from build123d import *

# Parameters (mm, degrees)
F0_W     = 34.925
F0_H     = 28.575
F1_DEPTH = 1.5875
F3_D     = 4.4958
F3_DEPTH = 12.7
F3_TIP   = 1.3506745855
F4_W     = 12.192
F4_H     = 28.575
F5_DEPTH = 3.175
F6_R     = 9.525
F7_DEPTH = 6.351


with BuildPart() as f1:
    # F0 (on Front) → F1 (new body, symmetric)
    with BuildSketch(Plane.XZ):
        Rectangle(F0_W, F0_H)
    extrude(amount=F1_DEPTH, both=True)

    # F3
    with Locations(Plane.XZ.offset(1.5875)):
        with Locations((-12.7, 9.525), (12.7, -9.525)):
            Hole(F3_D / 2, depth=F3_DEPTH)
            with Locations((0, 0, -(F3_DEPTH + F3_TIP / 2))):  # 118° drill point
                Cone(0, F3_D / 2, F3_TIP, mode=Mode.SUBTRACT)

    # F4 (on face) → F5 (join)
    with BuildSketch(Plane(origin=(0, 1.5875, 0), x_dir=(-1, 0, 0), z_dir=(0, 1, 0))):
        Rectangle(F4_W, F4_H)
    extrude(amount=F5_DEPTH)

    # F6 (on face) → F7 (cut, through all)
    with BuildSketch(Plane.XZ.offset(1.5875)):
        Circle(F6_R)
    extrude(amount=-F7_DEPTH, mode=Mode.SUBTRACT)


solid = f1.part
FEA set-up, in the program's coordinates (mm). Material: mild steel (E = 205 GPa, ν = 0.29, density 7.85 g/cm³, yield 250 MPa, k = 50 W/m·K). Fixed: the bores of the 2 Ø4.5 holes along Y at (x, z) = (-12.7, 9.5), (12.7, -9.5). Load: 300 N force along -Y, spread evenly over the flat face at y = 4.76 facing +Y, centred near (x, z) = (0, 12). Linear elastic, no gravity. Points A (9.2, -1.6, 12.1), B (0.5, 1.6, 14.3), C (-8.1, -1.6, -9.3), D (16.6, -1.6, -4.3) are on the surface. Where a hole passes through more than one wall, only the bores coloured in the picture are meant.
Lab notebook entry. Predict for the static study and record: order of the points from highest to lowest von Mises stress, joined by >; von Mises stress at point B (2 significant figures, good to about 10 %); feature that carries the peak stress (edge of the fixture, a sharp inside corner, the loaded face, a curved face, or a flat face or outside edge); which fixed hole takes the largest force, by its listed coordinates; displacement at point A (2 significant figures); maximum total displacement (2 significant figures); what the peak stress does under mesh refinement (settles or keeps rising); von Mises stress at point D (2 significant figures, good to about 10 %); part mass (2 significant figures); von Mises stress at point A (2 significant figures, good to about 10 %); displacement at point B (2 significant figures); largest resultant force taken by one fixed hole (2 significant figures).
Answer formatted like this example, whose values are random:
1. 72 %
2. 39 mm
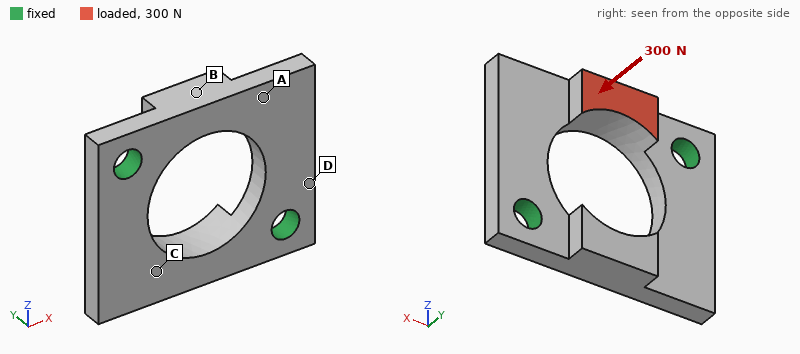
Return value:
1. D > A > B > C
2. 22 MPa
3. edge of the fixture
4. (-12.7, 9.5)
5. 21 µm
6. 27 µm
7. keeps rising
8. 48 MPa
9. 20 g
10. 31 MPa
11. 15 µm
12. 230 N
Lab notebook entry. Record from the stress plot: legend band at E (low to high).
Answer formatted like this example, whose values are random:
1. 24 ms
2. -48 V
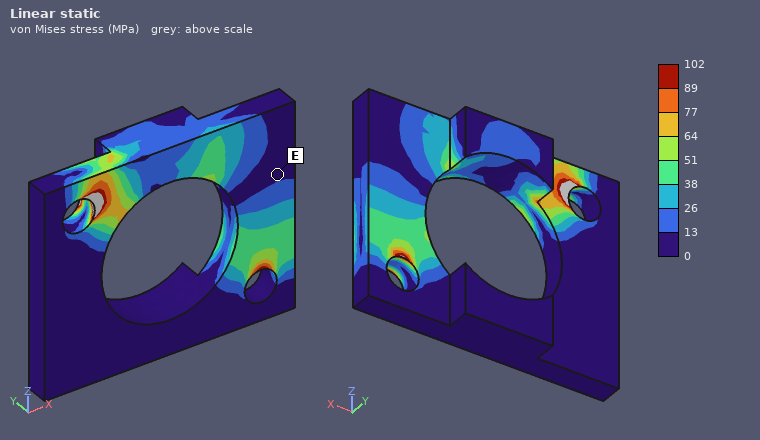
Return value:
1. 0 to 13 MPa
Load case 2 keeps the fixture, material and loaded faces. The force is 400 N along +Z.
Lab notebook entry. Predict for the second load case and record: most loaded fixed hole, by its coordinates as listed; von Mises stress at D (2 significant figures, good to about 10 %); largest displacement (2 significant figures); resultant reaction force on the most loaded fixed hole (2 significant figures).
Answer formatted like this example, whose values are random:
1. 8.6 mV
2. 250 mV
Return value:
1. (-12.7, 9.5)
2. 13 MPa
3. 17 µm
4. 240 N
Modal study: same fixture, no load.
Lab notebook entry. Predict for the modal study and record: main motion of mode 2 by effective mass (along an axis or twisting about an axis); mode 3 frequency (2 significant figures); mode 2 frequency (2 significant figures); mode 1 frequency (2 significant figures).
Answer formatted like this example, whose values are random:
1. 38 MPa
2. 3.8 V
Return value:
1. along Y
2. 22 kHz
3. 7000 Hz
4. 6600 Hz
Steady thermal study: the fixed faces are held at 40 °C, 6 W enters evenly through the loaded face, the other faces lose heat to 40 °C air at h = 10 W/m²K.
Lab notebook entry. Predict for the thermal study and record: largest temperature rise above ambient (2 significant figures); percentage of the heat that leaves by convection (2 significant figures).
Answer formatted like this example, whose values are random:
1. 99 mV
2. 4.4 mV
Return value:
1. 36 K
2. 3.0 %
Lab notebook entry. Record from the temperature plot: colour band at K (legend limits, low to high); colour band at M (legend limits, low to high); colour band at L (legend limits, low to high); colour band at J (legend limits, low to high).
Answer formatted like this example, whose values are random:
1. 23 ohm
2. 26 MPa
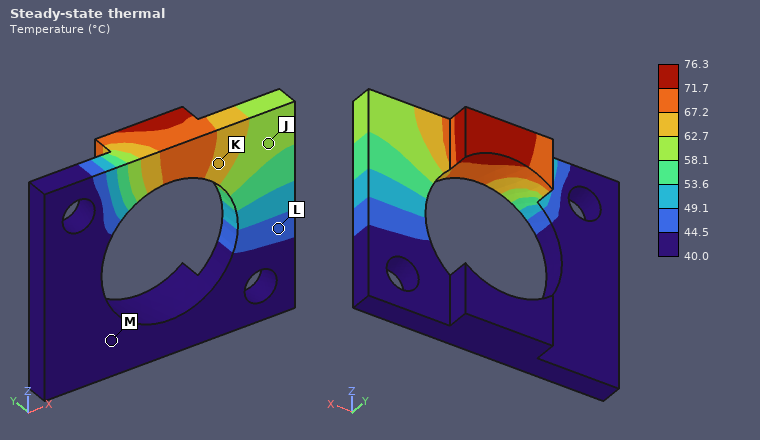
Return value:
1. 62.7 to 67.2 °C
2. 40.0 to 44.5 °C
3. 44.5 to 49.1 °C
4. 58.1 to 62.7 °C
